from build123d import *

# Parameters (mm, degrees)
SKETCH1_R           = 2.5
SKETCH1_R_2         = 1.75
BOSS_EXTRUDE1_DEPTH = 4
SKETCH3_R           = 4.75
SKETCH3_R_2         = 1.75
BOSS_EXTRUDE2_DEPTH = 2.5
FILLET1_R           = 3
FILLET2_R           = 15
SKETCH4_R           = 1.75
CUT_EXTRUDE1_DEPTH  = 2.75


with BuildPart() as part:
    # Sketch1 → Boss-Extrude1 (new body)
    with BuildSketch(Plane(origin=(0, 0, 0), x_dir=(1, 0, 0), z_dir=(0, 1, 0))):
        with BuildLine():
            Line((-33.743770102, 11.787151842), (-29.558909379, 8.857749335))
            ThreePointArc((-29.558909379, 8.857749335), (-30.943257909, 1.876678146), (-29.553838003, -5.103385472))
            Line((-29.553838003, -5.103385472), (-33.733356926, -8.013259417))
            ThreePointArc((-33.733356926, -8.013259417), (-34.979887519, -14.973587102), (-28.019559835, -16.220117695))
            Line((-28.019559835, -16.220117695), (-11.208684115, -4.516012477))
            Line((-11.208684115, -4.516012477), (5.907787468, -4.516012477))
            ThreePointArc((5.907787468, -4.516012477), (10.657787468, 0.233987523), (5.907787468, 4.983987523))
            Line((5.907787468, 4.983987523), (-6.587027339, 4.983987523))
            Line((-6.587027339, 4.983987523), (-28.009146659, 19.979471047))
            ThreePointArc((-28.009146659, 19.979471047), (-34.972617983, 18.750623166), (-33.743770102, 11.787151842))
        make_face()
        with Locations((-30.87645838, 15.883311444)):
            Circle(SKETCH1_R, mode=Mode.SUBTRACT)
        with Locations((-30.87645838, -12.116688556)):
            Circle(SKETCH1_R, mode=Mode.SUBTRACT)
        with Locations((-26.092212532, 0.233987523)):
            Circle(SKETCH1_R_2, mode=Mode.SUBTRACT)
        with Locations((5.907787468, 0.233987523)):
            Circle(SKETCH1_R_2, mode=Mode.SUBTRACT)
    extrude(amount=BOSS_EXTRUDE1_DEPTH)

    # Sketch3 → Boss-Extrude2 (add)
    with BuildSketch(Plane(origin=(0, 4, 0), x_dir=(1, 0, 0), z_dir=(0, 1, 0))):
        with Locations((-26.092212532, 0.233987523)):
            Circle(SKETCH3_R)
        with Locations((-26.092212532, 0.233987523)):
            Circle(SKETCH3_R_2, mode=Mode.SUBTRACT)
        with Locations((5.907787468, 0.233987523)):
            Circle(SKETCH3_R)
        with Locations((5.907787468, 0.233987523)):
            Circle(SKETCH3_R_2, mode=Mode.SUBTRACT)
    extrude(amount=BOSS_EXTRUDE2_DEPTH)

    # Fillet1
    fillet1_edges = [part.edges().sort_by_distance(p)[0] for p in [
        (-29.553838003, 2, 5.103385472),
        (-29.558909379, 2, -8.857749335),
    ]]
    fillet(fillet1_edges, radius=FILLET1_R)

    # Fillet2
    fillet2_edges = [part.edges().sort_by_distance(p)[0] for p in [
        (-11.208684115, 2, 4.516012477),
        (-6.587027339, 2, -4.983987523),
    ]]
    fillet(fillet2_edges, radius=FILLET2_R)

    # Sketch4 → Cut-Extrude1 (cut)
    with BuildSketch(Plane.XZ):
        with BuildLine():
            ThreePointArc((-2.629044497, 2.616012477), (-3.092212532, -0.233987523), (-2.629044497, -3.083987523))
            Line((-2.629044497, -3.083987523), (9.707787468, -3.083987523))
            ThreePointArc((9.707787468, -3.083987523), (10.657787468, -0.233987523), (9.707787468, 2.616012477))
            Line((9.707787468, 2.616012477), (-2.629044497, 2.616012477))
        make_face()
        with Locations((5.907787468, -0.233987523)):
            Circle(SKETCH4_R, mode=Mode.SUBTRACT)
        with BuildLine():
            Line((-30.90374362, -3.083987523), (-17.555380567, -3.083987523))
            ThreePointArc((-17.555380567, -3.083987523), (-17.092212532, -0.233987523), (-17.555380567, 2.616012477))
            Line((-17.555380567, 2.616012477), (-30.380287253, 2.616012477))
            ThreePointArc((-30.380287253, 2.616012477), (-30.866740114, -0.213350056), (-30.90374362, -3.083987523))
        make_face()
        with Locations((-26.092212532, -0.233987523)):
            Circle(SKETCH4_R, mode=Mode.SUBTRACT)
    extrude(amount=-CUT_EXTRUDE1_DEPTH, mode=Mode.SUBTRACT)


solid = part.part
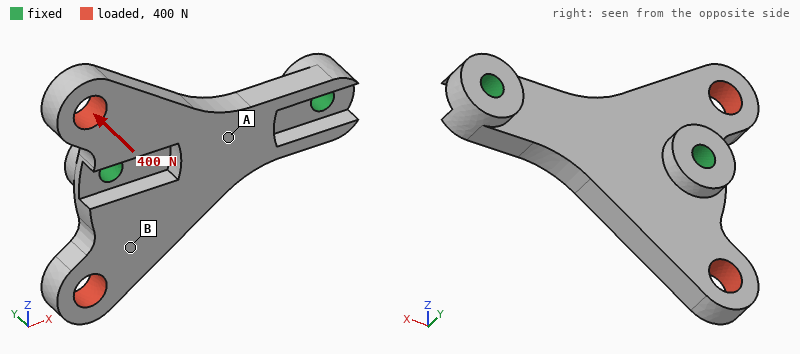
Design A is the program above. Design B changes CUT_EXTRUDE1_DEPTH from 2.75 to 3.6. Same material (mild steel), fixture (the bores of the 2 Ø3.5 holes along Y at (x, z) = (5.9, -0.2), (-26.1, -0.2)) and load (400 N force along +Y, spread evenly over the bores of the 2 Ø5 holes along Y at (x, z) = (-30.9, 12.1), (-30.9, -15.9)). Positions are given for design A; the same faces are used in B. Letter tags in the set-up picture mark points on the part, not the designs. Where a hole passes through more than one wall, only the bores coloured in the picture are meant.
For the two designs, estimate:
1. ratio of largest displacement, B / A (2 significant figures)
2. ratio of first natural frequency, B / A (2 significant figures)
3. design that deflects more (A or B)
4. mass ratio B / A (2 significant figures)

1.3
0.79
B
0.96
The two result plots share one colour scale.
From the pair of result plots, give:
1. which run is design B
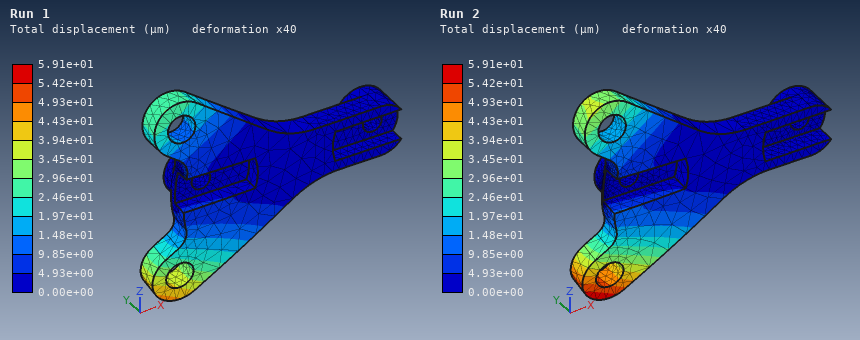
Run 2
